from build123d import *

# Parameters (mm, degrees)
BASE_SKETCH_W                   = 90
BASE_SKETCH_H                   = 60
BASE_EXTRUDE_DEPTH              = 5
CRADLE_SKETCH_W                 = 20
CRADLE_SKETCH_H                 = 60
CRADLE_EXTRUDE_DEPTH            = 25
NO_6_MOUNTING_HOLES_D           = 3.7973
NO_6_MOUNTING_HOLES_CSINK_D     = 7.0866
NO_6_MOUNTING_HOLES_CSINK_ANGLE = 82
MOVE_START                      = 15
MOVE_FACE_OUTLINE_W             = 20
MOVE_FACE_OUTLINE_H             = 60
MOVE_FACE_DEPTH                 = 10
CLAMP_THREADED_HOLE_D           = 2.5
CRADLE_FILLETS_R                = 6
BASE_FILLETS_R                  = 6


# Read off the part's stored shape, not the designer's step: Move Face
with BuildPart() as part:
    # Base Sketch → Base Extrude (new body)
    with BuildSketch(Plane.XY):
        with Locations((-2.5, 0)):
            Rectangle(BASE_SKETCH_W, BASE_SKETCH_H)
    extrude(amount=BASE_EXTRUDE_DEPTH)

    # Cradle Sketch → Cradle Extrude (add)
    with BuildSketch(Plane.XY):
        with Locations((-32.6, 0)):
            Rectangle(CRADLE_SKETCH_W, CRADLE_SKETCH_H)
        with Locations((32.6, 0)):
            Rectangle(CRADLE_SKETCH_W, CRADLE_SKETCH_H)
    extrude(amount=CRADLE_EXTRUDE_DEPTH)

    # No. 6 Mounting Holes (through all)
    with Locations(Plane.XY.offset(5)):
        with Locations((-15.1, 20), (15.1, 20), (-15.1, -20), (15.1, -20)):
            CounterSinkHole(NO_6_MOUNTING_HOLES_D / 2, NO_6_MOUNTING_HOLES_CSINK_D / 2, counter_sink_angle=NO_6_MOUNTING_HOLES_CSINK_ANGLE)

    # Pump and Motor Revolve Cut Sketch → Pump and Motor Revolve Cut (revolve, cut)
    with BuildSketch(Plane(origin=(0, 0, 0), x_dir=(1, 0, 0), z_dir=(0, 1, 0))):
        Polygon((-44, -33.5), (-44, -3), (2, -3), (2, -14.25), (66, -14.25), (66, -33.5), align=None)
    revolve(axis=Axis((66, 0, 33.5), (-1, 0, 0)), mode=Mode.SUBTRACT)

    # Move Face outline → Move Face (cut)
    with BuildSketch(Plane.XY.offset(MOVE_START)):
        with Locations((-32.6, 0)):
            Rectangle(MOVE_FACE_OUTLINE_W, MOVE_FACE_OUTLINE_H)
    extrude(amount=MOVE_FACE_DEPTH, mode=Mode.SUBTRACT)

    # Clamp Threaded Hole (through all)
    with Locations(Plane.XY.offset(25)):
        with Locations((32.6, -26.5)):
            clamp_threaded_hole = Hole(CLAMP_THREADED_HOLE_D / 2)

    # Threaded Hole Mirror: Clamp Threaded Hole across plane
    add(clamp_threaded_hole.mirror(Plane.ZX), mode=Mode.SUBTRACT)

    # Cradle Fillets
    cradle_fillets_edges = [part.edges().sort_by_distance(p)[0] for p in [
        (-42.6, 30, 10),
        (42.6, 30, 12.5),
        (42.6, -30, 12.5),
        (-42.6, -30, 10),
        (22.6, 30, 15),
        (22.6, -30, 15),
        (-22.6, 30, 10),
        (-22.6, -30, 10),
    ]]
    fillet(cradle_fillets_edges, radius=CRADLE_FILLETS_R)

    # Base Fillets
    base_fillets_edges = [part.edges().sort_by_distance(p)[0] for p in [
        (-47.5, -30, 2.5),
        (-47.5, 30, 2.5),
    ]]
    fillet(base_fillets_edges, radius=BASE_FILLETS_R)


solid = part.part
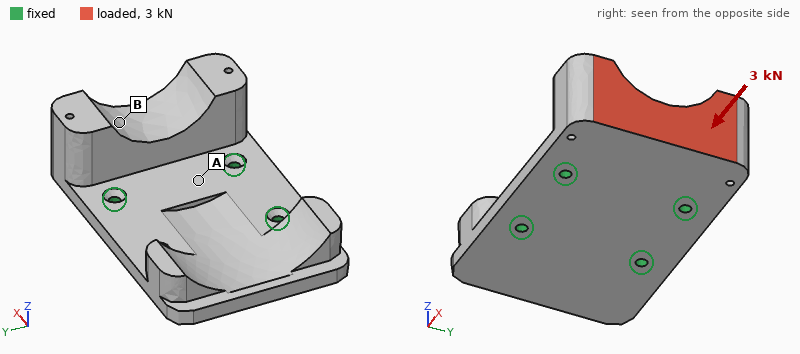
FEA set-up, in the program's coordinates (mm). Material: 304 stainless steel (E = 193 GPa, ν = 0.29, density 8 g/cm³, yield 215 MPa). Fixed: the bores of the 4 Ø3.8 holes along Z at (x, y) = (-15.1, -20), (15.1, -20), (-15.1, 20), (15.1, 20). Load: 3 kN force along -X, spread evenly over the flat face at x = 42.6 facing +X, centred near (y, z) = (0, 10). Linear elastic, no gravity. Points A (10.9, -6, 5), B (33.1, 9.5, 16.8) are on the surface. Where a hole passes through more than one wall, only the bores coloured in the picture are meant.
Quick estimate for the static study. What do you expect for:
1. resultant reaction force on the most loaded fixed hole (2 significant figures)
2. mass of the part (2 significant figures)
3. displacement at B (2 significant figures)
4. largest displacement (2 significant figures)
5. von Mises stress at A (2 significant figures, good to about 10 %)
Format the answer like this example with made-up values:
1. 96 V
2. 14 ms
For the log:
1. 820 N
2. 380 g
3. 56 µm
4. 89 µm
5. 48 MPa
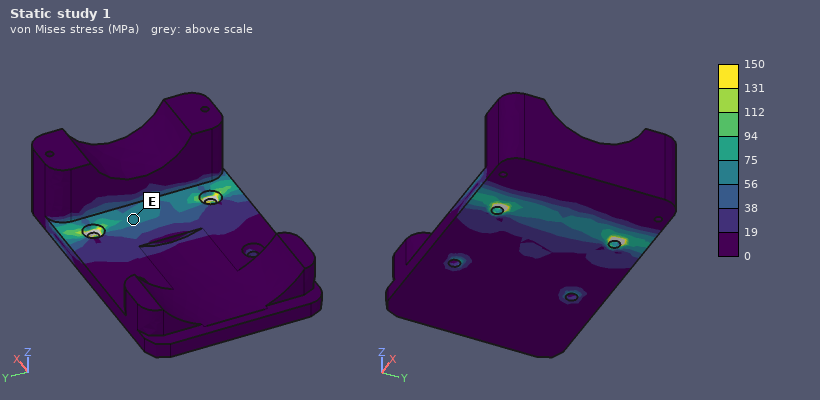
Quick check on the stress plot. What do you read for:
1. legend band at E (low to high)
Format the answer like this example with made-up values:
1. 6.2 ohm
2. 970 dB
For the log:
1. 56 to 75 MPa
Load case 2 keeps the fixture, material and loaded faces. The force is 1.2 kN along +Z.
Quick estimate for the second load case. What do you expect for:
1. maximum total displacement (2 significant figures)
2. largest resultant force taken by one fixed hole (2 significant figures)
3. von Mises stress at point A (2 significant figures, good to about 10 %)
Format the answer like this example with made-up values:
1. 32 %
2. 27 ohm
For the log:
1. 0.11 mm
2. 1.0 kN
3. 56 MPa
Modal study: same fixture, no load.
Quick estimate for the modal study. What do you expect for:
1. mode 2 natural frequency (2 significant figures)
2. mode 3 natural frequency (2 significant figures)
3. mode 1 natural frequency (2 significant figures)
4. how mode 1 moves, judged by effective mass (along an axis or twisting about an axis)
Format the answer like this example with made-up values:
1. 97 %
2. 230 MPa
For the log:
1. 2600 Hz
2. 4200 Hz
3. 1800 Hz
4. along Z
